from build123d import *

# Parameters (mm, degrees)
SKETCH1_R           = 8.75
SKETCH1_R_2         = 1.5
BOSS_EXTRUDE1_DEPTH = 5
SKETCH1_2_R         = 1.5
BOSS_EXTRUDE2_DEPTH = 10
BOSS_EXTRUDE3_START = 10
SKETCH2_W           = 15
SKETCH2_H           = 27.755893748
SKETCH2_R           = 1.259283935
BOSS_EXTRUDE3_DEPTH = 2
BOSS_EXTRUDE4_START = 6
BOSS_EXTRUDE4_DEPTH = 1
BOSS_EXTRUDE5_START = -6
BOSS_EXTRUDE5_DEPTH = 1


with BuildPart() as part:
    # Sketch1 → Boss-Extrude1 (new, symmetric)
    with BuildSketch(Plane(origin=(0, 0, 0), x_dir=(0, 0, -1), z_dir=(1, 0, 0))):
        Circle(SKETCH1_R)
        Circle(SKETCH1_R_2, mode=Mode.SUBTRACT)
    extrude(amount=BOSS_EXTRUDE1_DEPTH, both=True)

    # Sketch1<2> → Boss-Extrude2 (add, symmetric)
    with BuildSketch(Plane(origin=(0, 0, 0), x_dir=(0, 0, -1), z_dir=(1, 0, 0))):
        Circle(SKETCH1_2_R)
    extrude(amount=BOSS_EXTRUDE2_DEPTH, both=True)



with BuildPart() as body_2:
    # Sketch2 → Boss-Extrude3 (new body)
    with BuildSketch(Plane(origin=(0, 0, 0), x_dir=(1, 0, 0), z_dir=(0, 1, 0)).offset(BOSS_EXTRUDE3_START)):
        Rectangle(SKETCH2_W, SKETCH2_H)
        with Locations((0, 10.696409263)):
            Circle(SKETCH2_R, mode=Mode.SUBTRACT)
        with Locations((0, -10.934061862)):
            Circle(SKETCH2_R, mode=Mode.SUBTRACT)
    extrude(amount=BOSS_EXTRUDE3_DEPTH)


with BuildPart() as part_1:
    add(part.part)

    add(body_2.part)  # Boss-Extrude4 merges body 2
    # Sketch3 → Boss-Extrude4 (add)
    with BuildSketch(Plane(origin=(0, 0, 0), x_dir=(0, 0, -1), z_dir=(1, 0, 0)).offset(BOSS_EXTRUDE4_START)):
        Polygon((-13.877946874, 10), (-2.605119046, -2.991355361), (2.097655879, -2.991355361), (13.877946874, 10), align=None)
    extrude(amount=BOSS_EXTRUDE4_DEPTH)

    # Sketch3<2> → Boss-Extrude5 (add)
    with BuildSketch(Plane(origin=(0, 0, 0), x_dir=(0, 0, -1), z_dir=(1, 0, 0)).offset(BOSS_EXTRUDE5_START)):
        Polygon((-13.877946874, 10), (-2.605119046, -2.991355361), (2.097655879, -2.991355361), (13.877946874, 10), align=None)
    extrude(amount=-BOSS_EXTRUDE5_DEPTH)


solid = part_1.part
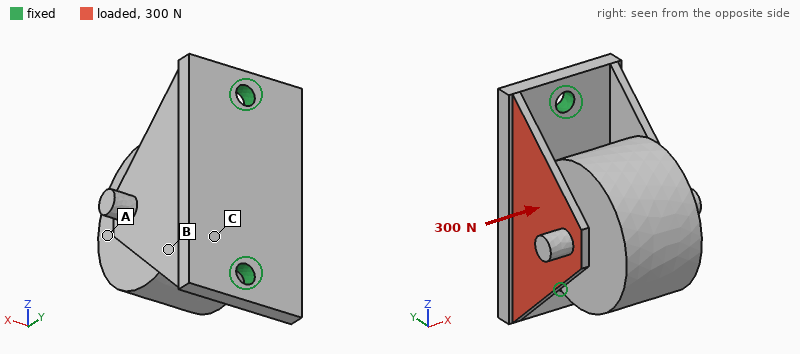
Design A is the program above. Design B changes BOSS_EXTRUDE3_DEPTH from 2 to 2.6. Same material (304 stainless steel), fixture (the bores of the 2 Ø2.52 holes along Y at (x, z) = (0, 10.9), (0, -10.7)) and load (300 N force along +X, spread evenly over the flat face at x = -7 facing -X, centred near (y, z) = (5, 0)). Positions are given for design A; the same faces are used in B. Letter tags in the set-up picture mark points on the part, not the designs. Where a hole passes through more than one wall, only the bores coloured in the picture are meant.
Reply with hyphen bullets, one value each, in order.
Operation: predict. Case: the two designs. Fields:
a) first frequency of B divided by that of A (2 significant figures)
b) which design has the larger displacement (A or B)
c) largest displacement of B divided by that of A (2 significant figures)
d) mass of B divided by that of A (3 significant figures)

- 1.1
- A
- 0.78
- 1.07
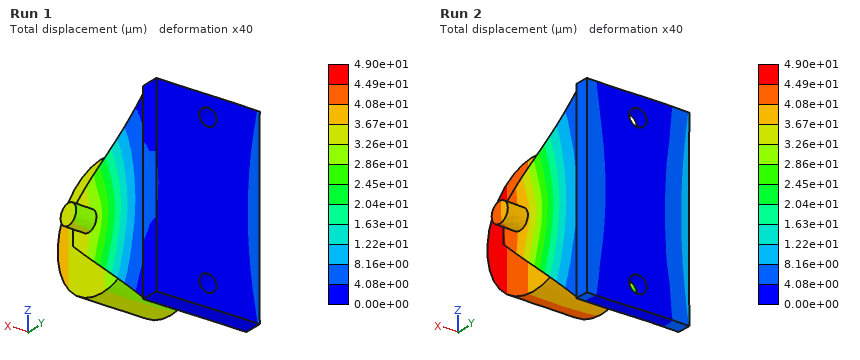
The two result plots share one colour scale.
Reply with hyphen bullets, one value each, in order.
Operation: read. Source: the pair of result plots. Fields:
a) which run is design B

- Run 1
